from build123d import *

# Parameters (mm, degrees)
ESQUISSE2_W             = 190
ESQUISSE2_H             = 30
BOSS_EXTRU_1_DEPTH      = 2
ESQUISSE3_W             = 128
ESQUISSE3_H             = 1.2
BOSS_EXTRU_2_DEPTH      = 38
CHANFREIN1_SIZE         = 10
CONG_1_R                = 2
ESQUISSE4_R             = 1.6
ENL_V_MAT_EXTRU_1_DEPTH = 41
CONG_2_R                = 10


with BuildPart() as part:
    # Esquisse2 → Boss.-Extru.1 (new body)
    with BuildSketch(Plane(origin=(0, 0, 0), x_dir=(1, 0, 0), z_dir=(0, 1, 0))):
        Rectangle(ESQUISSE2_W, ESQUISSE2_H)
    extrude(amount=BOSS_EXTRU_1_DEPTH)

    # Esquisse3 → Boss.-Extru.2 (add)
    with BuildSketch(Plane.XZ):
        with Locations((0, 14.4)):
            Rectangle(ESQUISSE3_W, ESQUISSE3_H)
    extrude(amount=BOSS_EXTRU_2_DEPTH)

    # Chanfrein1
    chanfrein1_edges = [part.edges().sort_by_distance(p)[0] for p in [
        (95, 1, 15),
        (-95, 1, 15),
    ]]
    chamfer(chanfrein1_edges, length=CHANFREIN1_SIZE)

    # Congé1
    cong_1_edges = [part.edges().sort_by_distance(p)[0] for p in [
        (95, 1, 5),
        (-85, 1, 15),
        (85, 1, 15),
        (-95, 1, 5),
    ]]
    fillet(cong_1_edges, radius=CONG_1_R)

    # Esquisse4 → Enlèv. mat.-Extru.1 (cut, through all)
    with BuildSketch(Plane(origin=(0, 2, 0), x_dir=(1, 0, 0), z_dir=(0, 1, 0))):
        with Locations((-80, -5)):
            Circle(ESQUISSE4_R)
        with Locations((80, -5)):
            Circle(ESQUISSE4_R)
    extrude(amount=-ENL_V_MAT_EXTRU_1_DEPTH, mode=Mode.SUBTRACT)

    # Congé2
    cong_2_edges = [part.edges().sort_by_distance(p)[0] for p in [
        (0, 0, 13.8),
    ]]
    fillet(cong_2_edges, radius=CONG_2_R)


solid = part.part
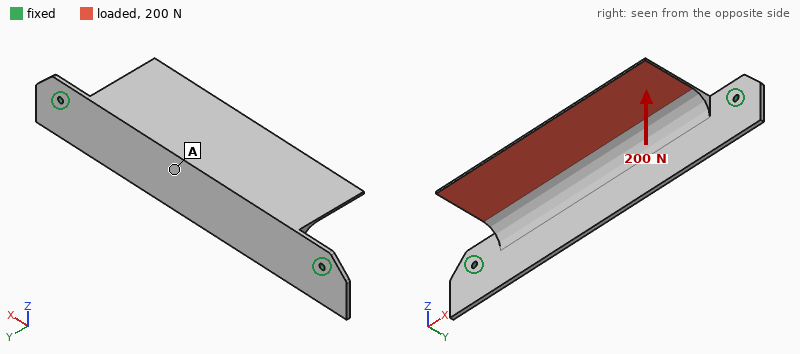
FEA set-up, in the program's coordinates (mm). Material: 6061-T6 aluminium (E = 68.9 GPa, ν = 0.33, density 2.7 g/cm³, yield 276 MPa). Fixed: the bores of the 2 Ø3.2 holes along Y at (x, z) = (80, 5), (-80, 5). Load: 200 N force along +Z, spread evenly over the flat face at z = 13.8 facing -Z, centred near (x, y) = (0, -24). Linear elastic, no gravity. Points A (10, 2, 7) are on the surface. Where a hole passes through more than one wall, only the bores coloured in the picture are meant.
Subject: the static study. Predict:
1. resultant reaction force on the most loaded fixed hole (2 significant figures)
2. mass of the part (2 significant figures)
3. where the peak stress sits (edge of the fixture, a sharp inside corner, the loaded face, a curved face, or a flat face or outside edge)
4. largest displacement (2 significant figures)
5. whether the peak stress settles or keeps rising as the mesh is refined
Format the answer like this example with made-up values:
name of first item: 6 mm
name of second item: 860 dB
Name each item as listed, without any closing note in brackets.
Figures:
resultant reaction force on the most loaded fixed hole: 100 N
mass of the part: 53 g
where the peak stress sits: edge of the fixture
largest displacement: 1.9 mm
whether the peak stress settles or keeps rising as the mesh is refined: keeps rising
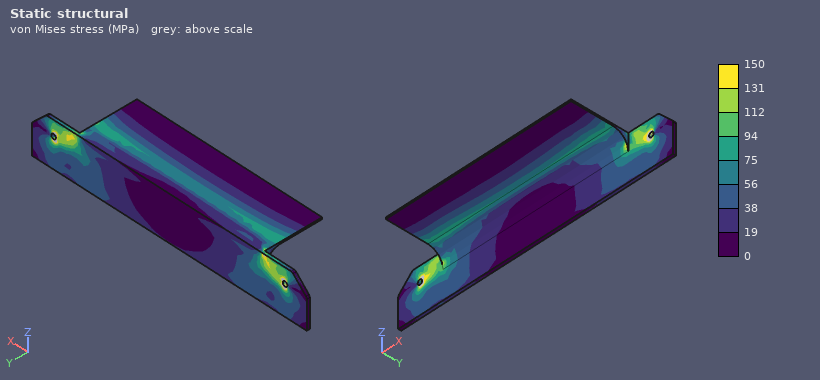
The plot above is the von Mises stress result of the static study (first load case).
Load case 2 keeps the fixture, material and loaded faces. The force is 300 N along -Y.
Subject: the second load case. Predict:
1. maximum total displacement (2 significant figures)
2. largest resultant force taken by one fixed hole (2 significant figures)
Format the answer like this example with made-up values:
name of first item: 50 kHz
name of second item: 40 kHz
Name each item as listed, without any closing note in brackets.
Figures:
maximum total displacement: 0.46 mm
largest resultant force taken by one fixed hole: 240 N
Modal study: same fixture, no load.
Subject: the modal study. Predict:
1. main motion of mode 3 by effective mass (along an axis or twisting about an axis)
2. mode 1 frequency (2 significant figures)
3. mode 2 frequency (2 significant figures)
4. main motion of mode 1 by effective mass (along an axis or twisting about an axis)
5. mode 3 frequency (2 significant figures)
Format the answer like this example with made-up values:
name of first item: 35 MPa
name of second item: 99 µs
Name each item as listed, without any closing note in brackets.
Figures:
main motion of mode 3 by effective mass: along Y
mode 1 frequency: 530 Hz
mode 2 frequency: 1000 Hz
main motion of mode 1 by effective mass: along Z
mode 3 frequency: 1100 Hz
